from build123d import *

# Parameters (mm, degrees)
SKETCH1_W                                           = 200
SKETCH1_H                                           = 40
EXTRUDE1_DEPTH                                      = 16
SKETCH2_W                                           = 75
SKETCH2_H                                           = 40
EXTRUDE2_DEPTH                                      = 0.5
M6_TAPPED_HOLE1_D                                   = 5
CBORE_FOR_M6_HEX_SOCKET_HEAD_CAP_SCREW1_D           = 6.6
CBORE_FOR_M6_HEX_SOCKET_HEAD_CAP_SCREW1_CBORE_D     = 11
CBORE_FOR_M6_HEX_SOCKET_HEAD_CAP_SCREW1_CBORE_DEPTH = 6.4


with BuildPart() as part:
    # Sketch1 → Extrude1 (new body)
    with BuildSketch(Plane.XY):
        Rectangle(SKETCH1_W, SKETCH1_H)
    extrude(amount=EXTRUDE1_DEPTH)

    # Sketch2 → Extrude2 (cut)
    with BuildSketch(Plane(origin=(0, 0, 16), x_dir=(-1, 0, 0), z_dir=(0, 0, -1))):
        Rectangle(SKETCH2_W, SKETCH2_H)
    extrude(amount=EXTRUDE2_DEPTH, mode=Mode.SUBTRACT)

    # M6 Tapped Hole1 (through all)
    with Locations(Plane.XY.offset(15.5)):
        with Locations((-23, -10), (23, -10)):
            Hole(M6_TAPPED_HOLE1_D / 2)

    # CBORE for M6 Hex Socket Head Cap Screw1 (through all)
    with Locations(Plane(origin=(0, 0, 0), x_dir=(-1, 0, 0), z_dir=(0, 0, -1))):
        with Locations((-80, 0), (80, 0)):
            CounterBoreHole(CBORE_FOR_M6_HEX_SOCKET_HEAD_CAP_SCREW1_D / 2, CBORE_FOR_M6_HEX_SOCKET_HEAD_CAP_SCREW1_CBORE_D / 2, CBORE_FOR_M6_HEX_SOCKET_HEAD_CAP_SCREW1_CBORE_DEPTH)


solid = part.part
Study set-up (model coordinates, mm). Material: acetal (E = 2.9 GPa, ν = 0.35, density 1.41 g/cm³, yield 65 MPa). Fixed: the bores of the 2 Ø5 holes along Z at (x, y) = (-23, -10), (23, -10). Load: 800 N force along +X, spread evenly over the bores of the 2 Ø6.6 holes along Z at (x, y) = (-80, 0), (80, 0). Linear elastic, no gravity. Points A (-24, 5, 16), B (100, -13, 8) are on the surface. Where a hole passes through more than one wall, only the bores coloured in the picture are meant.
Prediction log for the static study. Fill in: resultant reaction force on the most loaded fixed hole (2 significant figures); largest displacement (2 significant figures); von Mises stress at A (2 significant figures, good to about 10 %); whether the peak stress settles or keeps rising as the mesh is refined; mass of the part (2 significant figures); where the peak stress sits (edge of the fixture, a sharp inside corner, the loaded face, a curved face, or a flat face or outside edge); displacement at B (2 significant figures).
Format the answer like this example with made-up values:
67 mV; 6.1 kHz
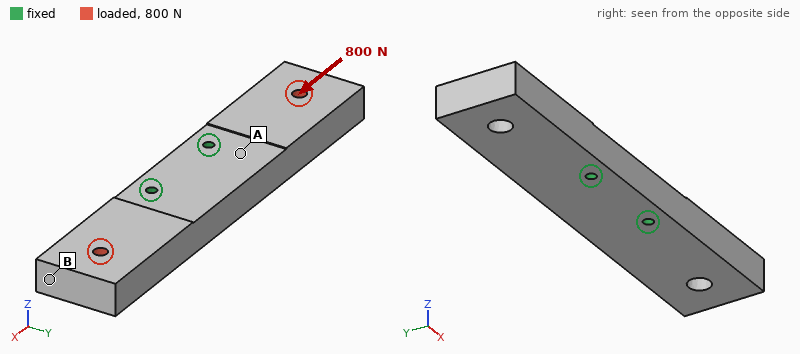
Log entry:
430 N; 0.12 mm; 1.1 MPa; keeps rising; 170 g; edge of the fixture; 0.11 mm
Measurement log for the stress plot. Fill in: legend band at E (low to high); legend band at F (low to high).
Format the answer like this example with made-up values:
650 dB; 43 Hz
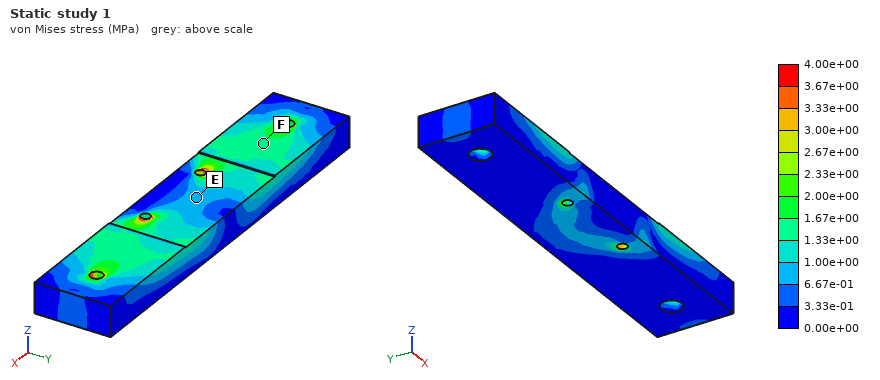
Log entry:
6.67e-01 to 1.00e+00 MPa; 1.33e+00 to 1.67e+00 MPa
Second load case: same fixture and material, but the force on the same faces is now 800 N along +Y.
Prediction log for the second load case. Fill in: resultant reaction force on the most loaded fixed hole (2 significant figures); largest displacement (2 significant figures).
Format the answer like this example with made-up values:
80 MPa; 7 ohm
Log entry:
820 N; 0.33 mm
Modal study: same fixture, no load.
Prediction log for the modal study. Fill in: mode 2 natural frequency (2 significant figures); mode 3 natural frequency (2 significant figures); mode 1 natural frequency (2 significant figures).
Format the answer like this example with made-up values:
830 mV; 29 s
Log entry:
530 Hz; 900 Hz; 520 Hz
